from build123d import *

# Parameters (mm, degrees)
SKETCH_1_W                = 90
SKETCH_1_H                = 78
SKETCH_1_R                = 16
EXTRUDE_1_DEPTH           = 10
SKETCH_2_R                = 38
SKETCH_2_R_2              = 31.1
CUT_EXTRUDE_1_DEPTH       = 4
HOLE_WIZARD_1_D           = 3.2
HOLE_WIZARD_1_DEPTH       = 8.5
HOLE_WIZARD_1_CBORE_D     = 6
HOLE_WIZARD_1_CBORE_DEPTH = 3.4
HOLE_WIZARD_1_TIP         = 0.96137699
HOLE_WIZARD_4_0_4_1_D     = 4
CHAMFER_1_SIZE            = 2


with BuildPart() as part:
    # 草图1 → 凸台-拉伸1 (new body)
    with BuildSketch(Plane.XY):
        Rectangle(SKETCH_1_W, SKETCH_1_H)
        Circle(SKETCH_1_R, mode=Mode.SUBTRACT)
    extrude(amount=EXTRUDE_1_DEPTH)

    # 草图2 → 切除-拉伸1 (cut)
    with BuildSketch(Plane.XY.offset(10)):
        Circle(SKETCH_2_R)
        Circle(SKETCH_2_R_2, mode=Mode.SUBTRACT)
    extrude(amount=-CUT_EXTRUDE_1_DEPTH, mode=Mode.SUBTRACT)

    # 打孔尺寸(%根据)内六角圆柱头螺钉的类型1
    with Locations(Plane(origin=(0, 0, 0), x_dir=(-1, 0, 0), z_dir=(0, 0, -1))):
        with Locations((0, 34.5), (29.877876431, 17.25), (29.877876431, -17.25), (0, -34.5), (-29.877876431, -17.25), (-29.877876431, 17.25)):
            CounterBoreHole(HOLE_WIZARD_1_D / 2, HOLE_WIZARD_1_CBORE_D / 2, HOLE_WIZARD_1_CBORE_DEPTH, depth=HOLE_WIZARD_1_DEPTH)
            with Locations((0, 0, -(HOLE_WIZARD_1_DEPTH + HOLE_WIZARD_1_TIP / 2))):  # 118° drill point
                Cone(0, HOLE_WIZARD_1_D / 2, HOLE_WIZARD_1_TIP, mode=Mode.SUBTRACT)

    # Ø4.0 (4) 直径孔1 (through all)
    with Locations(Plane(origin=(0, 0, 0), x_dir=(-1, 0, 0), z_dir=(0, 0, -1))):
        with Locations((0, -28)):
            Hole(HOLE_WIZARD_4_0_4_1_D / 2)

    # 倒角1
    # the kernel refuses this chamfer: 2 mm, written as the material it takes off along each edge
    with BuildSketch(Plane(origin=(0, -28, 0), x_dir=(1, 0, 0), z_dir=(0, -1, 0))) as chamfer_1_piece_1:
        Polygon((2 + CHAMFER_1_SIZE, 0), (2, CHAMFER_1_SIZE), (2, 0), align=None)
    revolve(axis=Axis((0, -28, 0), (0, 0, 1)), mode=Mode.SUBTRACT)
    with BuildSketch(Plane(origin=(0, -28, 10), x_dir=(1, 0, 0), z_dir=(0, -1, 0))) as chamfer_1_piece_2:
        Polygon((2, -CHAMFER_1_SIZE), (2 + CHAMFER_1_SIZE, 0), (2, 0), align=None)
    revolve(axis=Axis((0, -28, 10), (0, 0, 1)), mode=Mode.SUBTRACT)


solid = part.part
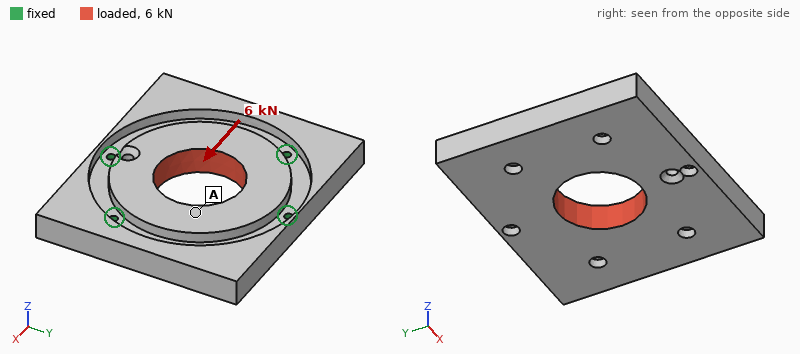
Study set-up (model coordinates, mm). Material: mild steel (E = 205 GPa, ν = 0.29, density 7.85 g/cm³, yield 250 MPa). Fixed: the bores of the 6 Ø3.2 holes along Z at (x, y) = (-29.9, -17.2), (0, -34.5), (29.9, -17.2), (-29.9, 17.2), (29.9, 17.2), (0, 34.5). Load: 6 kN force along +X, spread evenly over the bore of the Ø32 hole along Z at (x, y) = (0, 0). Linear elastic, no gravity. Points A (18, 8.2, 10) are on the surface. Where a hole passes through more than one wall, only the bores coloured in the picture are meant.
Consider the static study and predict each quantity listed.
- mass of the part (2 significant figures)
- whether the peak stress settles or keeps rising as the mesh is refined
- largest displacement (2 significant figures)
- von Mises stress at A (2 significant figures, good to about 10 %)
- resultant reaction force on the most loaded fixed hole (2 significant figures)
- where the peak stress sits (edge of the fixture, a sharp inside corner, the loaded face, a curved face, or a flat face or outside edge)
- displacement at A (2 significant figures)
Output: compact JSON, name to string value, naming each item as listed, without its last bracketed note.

{"mass of the part": "430 g", "whether the peak stress settles or keeps rising as the mesh is refined": "keeps rising", "largest displacement": "1.5 µm", "von Mises stress at A": "6.3 MPa", "resultant reaction force on the most loaded fixed hole": "1.2 kN", "where the peak stress sits": "edge of the fixture", "displacement at A": "1.3 µm"}
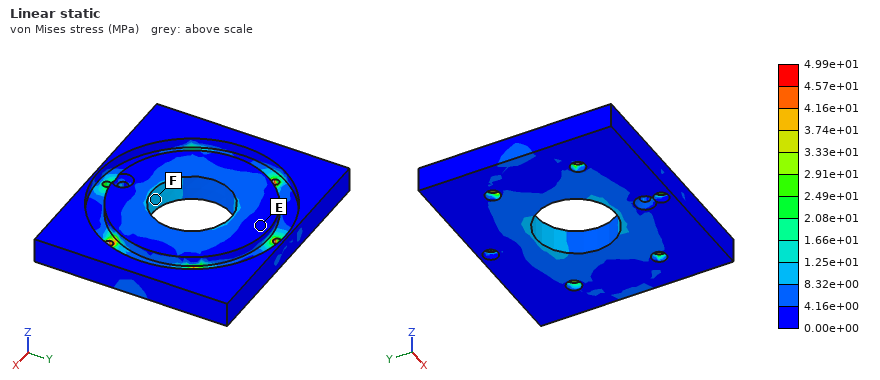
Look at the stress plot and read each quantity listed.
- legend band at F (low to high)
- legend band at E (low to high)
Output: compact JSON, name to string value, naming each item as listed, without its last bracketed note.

{"legend band at F": "8.32e+00 to 1.25e+01 MPa", "legend band at E": "0.00e+00 to 4.16e+00 MPa"}
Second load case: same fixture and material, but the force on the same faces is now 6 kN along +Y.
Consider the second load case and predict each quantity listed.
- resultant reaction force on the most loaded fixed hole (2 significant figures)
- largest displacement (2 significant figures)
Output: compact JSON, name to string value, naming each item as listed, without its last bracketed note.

{"resultant reaction force on the most loaded fixed hole": "1.2 kN", "largest displacement": "1.8 µm"}
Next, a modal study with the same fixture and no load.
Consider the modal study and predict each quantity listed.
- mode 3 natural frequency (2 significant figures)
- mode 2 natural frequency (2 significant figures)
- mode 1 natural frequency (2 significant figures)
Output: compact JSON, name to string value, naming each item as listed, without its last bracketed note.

{"mode 3 natural frequency": "7600 Hz", "mode 2 natural frequency": "7500 Hz", "mode 1 natural frequency": "7000 Hz"}
